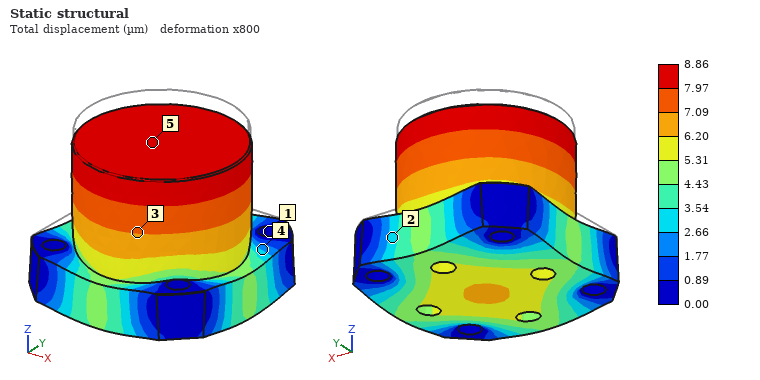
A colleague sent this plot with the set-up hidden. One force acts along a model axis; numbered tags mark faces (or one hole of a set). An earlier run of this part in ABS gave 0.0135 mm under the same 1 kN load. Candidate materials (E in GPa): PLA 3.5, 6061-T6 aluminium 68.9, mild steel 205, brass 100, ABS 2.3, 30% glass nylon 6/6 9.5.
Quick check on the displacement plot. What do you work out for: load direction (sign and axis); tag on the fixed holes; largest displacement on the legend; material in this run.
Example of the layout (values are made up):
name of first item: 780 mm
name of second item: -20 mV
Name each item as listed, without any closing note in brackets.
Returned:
load direction: -Z
tag on the fixed holes: 1
largest displacement on the legend: 8.86 µm
material in this run: PLA
